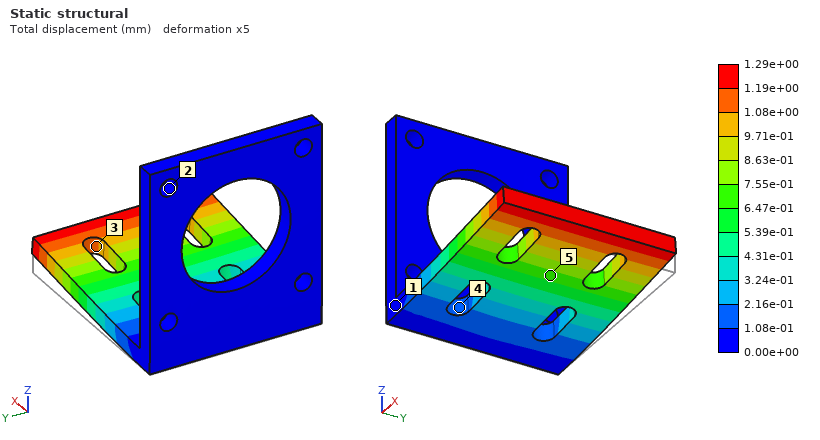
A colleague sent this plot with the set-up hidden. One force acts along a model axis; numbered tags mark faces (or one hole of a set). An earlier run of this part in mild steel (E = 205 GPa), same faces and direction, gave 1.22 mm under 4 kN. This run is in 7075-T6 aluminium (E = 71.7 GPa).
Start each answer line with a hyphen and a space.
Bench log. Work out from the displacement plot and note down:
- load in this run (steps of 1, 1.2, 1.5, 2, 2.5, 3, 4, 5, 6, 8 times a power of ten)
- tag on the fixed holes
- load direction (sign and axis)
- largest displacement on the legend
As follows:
- 1.5 kN
- 2
- +Z
- 1.29e+00 mm
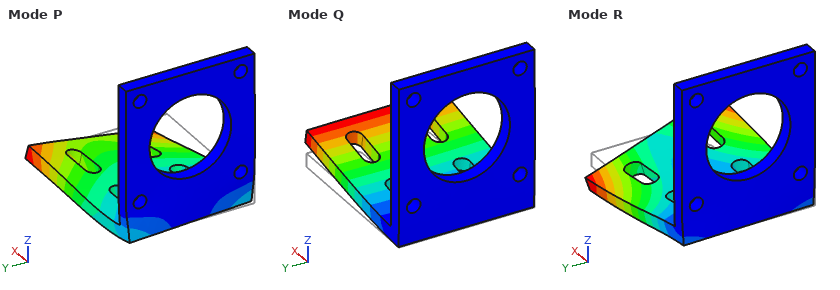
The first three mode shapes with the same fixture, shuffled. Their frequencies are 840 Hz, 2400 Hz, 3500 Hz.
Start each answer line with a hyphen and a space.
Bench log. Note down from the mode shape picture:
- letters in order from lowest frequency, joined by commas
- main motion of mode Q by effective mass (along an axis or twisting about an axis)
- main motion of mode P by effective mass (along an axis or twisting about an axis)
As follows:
- Q, R, P
- along Z
- along Y
